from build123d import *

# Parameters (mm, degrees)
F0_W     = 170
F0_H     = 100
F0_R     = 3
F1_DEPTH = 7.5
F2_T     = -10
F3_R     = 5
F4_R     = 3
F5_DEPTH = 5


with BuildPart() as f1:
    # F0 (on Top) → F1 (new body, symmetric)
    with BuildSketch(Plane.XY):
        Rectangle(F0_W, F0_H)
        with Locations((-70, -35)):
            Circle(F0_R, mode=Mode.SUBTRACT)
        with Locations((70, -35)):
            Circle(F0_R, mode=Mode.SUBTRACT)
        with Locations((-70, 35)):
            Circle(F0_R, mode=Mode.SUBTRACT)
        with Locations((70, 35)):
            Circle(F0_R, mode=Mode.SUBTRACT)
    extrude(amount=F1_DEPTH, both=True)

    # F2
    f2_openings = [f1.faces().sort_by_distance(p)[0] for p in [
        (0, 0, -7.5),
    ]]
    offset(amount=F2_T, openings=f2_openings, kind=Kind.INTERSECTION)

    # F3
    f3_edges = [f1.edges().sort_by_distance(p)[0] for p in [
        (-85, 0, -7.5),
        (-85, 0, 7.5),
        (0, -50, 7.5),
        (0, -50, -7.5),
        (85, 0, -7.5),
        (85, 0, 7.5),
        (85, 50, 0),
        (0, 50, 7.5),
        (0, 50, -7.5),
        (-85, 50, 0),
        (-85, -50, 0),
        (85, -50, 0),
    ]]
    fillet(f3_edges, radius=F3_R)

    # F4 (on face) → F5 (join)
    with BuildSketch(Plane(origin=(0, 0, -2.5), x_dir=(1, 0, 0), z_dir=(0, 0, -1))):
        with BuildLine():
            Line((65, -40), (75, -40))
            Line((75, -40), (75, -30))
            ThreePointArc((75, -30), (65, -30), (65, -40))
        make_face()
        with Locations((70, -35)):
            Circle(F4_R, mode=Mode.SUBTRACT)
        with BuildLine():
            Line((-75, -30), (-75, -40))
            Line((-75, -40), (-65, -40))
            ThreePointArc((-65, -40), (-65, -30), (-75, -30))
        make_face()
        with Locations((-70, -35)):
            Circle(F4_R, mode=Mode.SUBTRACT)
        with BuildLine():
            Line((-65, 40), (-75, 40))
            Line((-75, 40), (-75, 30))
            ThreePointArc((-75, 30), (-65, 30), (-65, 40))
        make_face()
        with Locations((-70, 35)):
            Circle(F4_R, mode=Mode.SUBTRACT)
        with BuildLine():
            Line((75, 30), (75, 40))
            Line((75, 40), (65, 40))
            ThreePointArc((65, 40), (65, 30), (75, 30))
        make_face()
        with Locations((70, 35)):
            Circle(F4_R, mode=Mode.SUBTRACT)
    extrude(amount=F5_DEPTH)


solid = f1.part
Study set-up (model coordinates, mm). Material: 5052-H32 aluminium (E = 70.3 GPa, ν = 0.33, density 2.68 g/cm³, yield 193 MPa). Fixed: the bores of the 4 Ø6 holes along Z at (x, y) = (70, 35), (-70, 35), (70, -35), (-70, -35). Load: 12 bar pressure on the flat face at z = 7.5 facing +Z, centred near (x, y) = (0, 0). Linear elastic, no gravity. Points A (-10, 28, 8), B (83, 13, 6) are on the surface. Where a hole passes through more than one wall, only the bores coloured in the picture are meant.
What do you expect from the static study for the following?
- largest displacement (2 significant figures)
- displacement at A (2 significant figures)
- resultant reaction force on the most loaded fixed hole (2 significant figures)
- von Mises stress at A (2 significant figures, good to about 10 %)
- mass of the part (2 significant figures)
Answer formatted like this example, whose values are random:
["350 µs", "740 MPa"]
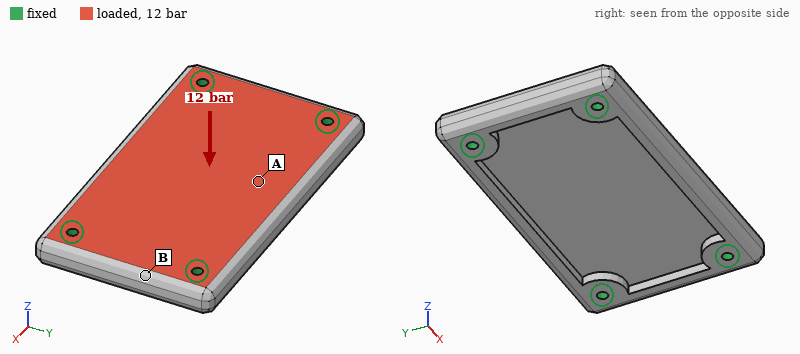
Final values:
["0.16 mm", "0.14 mm", "4.5 kN", "37 MPa", "520 g"]
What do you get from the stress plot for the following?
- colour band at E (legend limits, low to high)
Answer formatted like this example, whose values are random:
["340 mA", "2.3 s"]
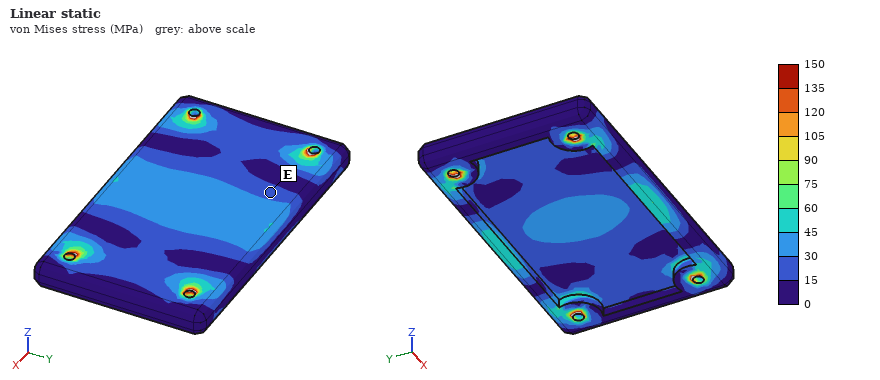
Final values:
["15 to 30 MPa"]
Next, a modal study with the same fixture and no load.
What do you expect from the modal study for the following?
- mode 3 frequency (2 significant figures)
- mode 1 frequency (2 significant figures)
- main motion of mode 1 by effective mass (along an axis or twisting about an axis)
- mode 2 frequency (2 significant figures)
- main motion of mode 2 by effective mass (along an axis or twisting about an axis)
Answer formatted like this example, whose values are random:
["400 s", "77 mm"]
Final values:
["7100 Hz", "2900 Hz", "along Z", "4100 Hz", "twisting about X"]
